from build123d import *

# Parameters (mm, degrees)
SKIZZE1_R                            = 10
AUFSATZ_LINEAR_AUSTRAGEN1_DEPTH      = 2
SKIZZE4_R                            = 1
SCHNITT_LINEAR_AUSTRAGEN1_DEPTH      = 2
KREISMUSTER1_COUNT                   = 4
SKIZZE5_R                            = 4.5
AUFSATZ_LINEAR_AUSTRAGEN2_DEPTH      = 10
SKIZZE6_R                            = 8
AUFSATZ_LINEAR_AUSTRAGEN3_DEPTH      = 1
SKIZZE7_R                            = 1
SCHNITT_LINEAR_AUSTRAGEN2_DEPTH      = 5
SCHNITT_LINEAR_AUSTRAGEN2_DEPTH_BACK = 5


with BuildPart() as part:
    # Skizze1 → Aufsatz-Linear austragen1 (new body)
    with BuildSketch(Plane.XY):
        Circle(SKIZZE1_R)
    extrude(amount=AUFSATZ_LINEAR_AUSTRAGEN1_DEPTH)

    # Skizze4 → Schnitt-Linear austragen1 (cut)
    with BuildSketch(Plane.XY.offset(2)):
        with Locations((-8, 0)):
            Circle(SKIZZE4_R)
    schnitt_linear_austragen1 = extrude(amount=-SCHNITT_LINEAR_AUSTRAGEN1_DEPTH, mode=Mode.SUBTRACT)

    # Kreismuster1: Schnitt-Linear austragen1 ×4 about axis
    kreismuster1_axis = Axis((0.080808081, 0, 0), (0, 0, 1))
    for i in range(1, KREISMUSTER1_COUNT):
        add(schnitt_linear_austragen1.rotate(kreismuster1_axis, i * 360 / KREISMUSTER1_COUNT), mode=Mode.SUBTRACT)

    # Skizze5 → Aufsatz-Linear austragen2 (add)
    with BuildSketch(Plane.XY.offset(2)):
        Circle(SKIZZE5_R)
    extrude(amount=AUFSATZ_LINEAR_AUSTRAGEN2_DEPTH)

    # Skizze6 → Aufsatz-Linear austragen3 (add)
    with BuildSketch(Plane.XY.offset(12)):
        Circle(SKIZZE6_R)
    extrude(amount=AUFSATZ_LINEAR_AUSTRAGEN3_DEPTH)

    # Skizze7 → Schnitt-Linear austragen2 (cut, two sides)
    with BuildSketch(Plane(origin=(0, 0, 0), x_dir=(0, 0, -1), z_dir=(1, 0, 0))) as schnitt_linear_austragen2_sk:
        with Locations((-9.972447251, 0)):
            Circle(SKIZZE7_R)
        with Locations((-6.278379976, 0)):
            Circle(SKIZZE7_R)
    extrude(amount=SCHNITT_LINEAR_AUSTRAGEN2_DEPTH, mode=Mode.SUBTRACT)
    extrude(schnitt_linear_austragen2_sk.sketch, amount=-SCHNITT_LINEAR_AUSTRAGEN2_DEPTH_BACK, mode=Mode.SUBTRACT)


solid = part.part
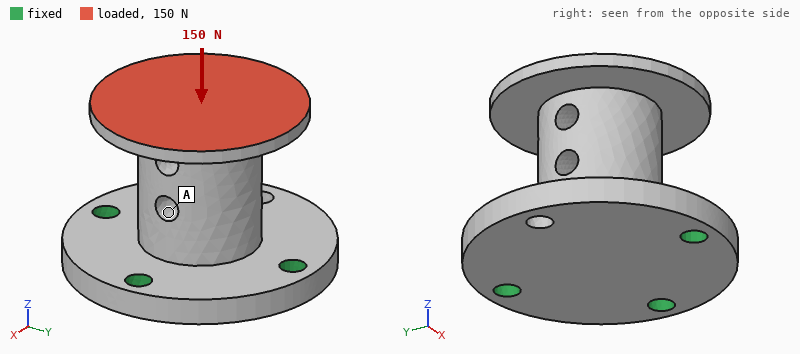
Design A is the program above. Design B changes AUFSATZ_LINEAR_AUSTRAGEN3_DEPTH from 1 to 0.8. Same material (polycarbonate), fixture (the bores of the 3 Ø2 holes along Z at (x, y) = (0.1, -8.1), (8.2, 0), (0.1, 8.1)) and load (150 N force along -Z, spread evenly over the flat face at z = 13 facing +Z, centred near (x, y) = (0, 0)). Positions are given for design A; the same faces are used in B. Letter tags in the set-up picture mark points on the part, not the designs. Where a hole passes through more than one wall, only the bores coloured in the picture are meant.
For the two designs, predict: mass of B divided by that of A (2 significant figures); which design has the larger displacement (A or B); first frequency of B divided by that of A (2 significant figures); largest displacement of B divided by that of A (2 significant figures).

0.97
B
1.1
1.3
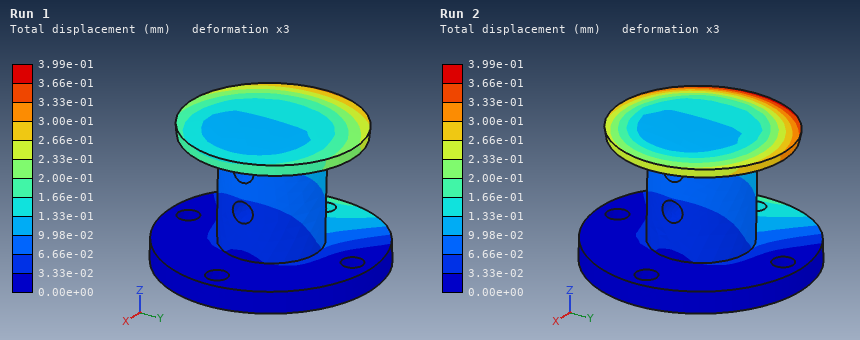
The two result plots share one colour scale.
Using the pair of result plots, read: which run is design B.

Run 2
